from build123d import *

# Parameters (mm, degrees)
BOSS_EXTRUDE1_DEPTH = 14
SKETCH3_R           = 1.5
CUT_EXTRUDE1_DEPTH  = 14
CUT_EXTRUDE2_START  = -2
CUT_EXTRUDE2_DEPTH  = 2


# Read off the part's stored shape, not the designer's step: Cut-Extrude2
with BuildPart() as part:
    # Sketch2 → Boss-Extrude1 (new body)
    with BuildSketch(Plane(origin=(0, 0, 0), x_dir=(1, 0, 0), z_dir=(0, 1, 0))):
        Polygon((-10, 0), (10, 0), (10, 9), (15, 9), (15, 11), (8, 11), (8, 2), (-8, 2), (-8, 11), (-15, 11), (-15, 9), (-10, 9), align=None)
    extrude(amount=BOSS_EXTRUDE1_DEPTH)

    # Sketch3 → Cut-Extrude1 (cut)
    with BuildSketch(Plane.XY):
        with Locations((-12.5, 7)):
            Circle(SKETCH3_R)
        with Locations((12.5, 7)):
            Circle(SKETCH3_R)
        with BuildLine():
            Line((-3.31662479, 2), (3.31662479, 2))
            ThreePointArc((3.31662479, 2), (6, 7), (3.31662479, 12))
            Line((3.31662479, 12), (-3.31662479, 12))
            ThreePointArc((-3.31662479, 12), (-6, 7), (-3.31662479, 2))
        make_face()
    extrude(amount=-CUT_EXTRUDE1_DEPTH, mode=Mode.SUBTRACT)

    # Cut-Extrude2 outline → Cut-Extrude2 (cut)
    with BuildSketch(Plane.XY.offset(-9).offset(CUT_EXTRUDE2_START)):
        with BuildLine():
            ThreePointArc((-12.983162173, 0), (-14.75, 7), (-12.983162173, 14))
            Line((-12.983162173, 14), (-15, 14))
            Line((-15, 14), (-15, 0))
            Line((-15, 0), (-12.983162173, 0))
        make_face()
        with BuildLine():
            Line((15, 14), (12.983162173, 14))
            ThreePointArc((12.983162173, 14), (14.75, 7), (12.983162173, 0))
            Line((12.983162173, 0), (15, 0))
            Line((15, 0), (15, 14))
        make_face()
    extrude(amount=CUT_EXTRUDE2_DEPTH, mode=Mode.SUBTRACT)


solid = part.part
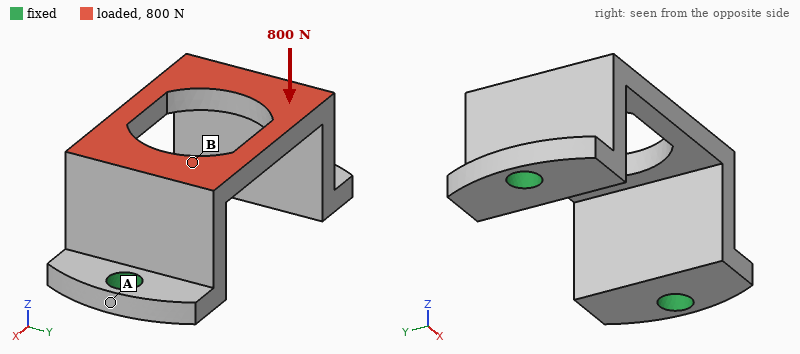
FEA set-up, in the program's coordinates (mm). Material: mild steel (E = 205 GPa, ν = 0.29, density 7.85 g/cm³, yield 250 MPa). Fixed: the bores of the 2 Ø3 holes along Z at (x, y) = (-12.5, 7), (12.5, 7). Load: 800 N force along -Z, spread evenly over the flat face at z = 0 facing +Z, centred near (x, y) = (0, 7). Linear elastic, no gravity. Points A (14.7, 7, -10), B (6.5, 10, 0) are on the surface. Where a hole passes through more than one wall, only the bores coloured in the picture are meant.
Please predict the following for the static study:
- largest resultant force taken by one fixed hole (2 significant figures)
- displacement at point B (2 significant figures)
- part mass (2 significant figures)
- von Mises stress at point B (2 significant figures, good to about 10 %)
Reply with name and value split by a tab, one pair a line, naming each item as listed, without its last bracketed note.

largest resultant force taken by one fixed hole	430 N
displacement at point B	5.4 µm
part mass	8.3 g
von Mises stress at point B	33 MPa
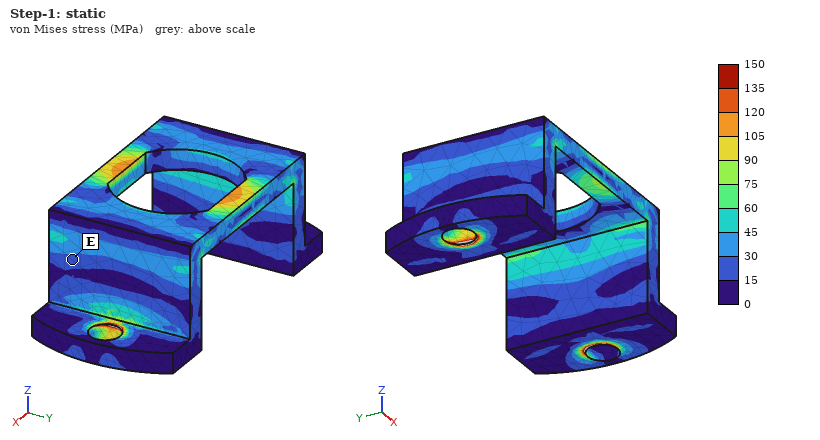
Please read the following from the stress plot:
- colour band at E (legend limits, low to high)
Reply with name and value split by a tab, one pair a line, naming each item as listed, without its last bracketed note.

colour band at E	15 to 30 MPa
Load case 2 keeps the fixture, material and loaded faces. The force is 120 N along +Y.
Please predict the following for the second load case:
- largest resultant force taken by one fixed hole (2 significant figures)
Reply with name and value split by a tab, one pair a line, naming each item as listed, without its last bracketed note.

largest resultant force taken by one fixed hole	60 N
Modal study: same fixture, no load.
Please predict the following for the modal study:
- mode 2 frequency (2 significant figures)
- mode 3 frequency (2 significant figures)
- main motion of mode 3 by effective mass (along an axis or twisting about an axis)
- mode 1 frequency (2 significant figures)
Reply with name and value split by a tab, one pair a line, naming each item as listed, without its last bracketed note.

mode 2 frequency	11 kHz
mode 3 frequency	14 kHz
main motion of mode 3 by effective mass	twisting about Z
mode 1 frequency	11 kHz
